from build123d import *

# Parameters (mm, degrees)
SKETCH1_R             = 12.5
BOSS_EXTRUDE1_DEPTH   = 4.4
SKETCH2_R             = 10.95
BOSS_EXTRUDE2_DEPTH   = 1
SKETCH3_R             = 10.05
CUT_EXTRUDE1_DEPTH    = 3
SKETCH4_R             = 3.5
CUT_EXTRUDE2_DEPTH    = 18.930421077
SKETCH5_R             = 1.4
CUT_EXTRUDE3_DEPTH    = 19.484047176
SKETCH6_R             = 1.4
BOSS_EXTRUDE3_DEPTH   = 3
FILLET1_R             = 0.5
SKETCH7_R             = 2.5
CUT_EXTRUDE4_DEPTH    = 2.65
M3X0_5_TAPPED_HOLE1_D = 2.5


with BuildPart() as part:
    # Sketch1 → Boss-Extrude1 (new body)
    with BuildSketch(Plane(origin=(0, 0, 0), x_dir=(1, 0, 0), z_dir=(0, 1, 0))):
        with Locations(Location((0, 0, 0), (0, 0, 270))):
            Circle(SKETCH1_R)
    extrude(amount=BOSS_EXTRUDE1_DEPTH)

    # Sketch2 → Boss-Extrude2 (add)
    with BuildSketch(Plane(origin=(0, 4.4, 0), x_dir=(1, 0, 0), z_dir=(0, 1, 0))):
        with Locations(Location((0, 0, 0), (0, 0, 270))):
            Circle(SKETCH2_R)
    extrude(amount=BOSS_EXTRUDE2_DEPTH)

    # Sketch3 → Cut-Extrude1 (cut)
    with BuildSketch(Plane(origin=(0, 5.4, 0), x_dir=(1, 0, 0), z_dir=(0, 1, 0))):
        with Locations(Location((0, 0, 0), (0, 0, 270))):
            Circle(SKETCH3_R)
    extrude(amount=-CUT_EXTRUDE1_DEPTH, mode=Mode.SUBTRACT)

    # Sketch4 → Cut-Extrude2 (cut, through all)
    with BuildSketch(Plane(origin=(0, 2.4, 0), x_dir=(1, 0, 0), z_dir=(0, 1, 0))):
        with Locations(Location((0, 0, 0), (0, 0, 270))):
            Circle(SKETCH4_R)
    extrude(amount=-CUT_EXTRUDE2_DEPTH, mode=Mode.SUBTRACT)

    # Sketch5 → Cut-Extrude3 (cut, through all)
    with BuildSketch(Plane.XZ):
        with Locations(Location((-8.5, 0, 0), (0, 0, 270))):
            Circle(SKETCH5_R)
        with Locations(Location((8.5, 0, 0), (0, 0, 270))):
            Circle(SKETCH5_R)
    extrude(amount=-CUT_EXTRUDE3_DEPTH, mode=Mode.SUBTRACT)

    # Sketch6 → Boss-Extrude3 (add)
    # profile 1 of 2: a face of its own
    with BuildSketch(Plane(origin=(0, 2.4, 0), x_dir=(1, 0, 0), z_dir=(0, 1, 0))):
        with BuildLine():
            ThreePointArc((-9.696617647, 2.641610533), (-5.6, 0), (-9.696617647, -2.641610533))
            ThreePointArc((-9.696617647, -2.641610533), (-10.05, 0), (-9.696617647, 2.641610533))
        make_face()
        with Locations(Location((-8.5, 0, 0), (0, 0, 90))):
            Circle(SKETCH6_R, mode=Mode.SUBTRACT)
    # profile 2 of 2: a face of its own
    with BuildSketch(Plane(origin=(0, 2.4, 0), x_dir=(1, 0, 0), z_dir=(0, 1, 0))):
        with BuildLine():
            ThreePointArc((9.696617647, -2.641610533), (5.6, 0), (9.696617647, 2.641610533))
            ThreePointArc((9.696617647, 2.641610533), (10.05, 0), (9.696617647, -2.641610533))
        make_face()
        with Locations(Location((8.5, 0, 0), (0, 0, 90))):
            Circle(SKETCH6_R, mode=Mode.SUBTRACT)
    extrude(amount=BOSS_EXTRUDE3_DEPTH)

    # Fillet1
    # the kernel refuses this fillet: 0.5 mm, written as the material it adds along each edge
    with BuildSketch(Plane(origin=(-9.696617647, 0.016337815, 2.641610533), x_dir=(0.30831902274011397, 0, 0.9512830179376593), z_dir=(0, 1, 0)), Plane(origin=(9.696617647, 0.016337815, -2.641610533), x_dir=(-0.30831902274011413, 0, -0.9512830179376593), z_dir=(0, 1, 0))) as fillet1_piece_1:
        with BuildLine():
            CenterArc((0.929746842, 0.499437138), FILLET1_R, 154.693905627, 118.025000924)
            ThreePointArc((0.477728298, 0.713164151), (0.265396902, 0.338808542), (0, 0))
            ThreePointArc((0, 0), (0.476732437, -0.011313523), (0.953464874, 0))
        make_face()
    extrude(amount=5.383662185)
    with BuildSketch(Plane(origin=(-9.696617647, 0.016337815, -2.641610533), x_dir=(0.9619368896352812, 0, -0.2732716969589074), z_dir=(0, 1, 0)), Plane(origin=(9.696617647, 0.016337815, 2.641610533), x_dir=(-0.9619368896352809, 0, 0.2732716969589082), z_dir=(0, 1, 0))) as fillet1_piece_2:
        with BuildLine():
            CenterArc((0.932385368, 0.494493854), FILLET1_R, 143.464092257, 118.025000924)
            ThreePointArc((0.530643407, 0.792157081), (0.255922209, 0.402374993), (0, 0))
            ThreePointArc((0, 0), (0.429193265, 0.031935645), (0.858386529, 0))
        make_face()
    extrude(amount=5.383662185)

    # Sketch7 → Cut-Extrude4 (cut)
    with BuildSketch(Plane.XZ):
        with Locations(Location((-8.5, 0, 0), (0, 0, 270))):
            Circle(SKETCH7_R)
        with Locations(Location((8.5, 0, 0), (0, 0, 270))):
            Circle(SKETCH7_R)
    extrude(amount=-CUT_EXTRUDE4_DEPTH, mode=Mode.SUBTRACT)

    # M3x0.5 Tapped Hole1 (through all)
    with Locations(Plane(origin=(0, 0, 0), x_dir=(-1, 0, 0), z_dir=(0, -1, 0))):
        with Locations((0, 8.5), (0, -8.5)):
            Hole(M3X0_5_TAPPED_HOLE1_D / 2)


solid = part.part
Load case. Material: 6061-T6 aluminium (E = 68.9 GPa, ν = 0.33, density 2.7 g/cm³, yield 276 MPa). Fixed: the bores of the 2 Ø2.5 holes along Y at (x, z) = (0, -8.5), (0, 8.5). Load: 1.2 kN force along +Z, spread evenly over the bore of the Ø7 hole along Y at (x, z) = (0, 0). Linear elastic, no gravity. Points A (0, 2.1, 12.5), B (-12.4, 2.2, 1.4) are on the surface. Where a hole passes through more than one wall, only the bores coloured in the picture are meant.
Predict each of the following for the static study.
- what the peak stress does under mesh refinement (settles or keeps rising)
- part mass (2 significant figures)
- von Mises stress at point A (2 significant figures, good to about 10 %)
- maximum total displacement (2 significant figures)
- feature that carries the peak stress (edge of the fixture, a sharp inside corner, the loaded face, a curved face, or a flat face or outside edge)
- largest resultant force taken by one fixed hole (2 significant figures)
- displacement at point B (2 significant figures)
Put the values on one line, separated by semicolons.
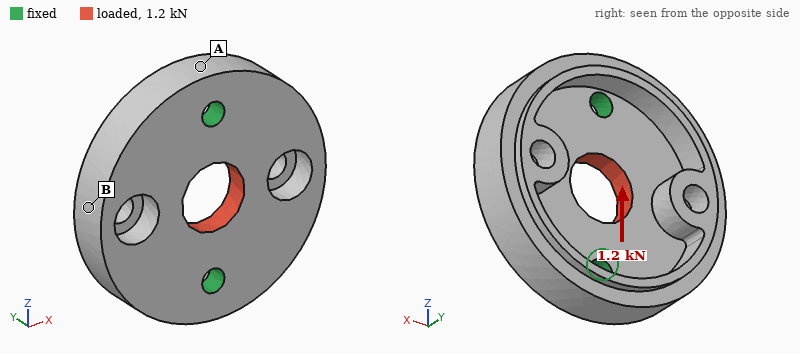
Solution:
keeps rising; 3.9 g; 15 MPa; 3.8 µm; edge of the fixture; 600 N; 2.0 µm
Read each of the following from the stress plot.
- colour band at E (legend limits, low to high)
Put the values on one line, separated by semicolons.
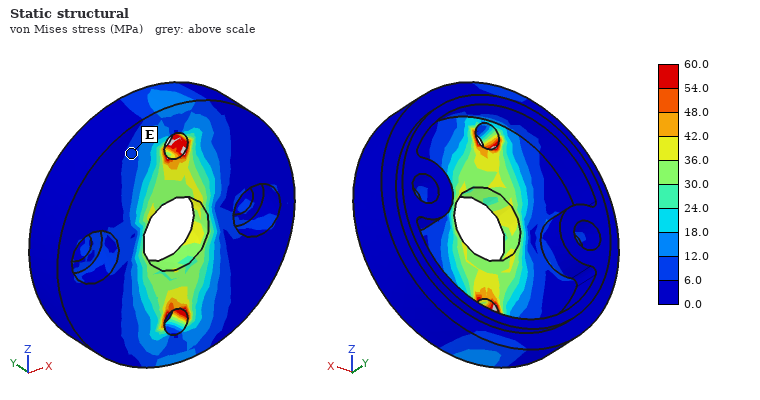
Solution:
6.0 to 12.0 MPa
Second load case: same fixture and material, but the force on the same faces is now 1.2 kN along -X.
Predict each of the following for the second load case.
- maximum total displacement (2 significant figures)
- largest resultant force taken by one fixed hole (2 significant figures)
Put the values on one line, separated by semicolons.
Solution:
5.8 µm; 600 N
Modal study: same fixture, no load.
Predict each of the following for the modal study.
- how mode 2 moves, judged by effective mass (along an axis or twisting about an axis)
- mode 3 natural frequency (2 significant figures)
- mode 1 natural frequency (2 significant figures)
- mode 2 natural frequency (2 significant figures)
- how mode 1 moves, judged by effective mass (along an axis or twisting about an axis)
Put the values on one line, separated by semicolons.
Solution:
along Y; 30 kHz; 13 kHz; 17 kHz; twisting about Z
